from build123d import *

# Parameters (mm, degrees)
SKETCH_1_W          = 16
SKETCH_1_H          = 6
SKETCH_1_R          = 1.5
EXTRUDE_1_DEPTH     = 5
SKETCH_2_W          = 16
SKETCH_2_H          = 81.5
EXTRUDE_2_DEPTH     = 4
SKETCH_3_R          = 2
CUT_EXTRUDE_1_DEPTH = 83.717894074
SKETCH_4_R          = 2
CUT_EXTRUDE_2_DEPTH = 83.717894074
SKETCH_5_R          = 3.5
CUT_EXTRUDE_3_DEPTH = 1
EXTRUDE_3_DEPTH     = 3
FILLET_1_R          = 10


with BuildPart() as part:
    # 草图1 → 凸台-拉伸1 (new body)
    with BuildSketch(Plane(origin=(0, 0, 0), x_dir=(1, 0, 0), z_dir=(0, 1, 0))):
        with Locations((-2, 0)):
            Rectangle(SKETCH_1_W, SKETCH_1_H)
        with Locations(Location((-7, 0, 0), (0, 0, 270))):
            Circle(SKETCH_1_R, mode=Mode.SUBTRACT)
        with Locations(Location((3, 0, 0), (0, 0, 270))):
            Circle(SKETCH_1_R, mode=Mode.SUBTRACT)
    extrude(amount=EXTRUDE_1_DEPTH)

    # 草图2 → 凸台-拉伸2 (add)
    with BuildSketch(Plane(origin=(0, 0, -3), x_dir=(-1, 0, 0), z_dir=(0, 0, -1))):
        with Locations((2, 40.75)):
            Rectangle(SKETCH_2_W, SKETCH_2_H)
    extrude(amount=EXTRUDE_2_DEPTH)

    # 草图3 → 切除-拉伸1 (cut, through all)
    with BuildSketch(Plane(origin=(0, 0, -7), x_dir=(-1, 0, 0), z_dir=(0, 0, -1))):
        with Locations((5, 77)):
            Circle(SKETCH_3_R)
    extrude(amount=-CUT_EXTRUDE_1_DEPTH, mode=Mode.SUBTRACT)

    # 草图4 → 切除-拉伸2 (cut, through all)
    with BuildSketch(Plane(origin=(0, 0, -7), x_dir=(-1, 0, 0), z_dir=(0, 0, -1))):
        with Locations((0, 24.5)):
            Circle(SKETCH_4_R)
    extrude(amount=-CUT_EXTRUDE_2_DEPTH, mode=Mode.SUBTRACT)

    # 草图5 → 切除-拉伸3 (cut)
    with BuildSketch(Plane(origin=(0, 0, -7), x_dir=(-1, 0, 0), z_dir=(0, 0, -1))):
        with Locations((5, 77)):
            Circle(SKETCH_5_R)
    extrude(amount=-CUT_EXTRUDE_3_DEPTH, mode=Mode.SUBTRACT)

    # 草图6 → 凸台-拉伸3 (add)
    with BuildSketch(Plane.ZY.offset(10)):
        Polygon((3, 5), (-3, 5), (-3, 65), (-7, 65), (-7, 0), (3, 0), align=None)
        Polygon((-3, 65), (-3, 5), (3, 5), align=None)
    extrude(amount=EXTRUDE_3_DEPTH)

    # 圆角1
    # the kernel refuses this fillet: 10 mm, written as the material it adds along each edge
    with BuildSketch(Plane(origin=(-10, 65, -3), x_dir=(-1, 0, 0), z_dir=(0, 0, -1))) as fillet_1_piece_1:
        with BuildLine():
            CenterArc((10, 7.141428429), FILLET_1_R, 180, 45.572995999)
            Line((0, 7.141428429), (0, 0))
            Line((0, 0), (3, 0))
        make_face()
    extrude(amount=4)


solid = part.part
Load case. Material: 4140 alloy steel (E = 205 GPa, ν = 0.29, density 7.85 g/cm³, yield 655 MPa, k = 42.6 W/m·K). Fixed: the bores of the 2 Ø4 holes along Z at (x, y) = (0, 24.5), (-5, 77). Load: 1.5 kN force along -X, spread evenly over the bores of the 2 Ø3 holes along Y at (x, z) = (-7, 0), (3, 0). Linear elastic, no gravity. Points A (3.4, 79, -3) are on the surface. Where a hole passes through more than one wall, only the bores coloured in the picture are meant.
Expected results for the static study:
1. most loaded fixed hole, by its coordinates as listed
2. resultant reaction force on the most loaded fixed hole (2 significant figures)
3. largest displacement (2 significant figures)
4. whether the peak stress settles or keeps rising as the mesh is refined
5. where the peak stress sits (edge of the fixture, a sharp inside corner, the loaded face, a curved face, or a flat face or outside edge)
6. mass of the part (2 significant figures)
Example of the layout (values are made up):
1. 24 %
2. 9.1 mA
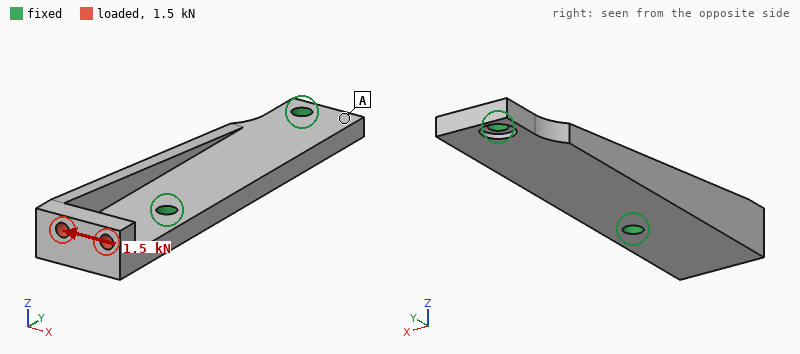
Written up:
1. (0, 24.5)
2. 2.0 kN
3. 93 µm
4. keeps rising
5. edge of the fixture
6. 54 g
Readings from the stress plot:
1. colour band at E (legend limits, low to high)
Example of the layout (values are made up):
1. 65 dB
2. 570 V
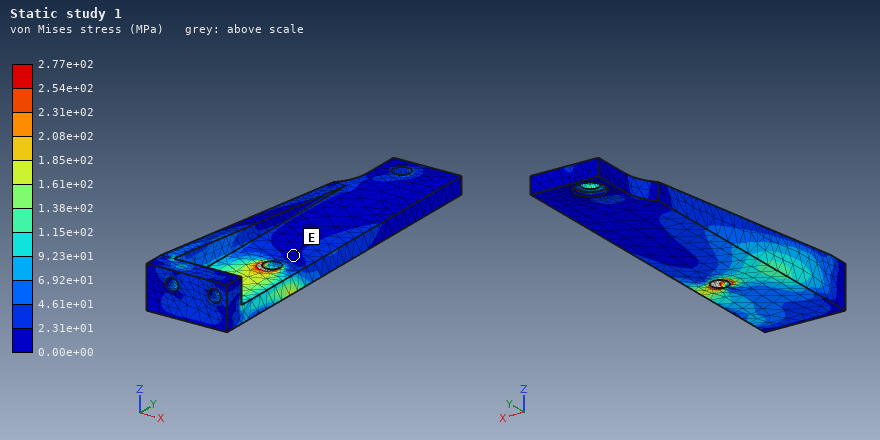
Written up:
1. 0.00e+00 to 2.31e+01 MPa
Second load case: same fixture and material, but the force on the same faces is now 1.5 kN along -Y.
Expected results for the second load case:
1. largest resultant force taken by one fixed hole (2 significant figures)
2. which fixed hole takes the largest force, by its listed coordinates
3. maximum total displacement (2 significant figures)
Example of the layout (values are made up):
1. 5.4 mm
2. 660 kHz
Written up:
1. 1.3 kN
2. (0, 24.5)
3. 69 µm
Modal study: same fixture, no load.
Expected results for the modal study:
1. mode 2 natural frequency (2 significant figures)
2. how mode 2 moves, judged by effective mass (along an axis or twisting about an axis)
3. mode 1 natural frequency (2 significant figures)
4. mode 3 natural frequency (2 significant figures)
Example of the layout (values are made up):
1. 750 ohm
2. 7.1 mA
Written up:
1. 7100 Hz
2. along Z
3. 4500 Hz
4. 8300 Hz
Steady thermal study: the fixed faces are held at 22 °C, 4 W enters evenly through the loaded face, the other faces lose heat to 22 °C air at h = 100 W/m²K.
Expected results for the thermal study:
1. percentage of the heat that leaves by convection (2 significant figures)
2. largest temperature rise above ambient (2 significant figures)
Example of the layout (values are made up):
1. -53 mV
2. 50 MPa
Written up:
1. 48 %
2. 22 K
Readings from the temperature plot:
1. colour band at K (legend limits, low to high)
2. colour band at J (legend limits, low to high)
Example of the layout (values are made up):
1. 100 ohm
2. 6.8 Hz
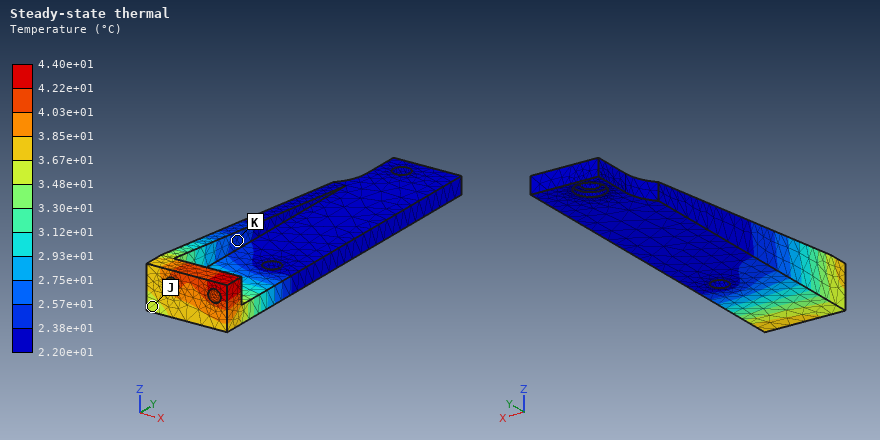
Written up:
1. 2.38e+01 to 2.57e+01 °C
2. 3.48e+01 to 3.67e+01 °C
